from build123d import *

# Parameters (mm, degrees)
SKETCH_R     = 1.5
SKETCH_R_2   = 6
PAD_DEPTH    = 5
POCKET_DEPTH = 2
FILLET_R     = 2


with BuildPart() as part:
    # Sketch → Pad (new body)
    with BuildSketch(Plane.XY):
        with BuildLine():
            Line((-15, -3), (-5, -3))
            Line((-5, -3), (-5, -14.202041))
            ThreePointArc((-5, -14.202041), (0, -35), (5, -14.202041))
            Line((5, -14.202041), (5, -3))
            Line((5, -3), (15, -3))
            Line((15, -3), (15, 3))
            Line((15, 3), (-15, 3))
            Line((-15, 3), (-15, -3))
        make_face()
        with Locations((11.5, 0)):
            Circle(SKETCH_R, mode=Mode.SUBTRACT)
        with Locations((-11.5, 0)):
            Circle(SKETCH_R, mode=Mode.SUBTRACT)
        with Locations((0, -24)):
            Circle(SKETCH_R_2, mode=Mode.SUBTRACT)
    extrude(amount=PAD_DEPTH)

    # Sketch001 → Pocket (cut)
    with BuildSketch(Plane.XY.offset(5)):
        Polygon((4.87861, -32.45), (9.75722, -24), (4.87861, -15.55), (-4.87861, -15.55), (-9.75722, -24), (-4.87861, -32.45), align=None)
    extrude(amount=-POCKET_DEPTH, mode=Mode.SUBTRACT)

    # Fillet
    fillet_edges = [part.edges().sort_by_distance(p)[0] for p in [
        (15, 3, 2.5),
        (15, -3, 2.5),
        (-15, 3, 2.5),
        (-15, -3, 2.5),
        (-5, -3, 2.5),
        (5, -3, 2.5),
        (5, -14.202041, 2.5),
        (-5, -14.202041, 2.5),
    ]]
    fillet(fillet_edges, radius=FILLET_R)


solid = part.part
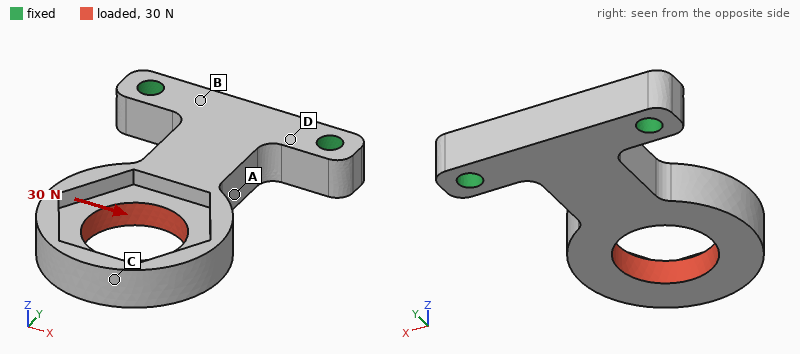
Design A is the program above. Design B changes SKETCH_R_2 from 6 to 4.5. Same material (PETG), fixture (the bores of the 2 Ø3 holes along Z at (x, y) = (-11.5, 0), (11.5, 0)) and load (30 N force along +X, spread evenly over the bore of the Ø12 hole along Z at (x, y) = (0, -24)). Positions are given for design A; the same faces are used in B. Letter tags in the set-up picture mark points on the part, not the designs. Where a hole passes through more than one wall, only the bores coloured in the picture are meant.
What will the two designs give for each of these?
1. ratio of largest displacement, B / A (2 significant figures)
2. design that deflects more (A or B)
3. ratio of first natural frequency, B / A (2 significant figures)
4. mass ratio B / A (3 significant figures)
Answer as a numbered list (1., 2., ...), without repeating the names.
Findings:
1. 0.86
2. A
3. 0.96
4. 1.06
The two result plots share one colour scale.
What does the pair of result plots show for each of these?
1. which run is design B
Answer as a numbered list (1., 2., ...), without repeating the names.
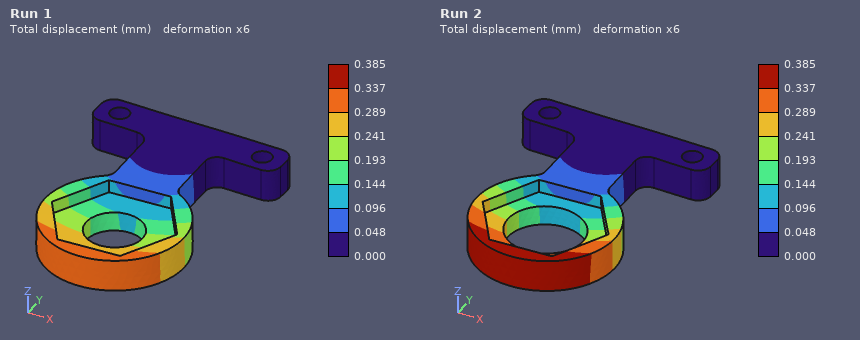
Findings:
1. Run 1
